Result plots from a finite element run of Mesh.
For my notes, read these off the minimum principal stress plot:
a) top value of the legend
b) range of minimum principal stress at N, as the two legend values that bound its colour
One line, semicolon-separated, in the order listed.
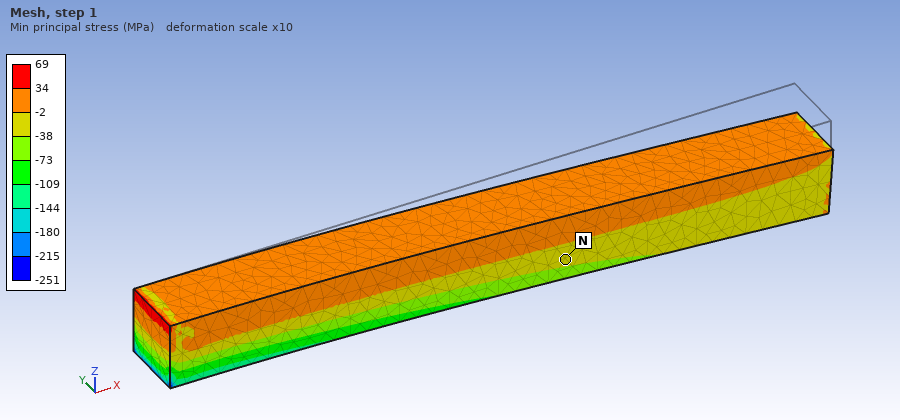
69 MPa; -38 to -2 MPa
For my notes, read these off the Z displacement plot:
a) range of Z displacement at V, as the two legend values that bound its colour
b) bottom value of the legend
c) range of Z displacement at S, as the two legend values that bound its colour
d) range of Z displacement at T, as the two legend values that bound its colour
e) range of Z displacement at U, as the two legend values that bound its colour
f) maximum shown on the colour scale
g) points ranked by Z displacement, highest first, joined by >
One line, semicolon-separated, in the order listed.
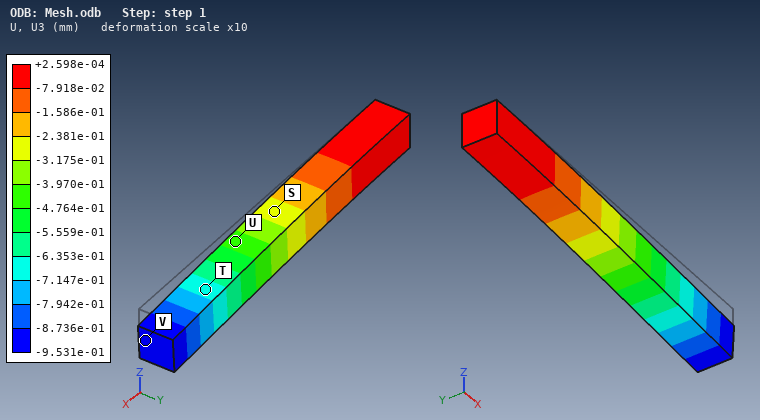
-9.531e-01 to -8.736e-01 mm; -9.531e-01 mm; -3.175e-01 to -2.381e-01 mm; -7.147e-01 to -6.353e-01 mm; -4.764e-01 to -3.970e-01 mm; +2.598e-04 mm; S > U > T > V
